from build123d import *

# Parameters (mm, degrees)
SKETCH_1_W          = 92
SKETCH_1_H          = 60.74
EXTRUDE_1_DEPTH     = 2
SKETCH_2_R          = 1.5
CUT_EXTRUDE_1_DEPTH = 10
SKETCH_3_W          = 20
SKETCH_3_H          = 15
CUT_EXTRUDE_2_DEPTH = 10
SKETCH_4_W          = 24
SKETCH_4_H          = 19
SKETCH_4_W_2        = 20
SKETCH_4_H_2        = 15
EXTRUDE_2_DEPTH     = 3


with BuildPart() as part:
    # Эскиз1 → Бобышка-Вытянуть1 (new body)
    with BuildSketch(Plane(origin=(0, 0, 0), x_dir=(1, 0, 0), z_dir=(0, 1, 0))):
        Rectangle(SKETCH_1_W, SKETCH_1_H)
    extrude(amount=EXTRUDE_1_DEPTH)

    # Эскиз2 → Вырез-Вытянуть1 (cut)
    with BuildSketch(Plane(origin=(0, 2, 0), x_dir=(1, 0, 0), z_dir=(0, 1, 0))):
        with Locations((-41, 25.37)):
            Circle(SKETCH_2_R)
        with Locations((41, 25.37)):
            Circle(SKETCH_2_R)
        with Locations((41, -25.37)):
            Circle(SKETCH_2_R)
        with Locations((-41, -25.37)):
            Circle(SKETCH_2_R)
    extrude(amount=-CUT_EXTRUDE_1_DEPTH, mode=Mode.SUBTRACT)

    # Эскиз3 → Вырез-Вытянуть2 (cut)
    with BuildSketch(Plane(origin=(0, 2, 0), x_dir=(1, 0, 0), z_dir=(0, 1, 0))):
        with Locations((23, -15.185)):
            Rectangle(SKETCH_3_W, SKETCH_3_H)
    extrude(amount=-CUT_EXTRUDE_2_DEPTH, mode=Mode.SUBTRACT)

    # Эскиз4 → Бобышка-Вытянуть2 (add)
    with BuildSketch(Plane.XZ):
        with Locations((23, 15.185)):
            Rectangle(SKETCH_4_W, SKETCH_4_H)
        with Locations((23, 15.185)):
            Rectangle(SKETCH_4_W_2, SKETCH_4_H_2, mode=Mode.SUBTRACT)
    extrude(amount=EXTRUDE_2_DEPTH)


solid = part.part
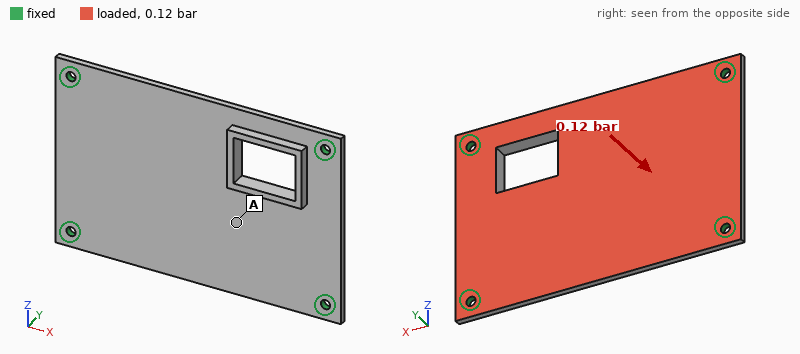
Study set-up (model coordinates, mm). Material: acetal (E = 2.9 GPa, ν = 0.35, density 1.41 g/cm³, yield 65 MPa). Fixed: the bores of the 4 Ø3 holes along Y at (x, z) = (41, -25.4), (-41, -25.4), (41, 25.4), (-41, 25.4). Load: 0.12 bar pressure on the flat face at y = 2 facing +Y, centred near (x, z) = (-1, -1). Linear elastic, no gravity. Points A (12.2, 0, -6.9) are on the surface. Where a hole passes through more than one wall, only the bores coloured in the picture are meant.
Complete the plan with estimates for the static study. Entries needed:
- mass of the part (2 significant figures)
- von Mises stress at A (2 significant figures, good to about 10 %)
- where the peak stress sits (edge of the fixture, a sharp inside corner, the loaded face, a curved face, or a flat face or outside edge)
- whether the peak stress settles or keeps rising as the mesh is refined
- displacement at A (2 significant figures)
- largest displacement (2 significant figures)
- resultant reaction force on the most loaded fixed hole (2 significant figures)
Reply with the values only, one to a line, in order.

15 g
3.8 MPa
edge of the fixture
keeps rising
0.85 mm
0.99 mm
17 N
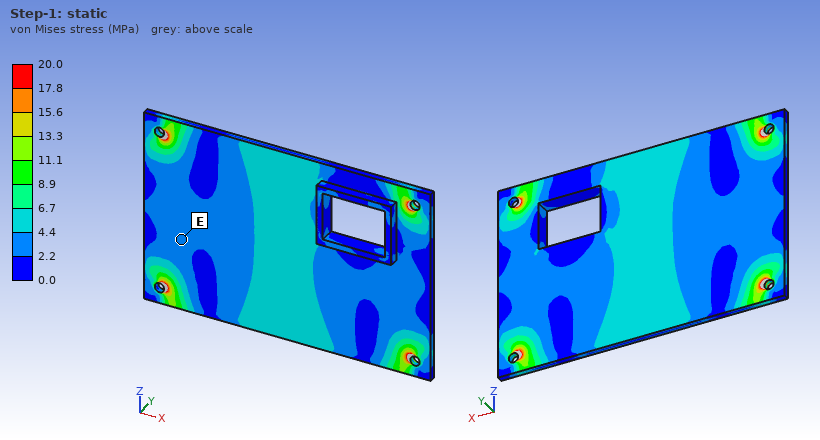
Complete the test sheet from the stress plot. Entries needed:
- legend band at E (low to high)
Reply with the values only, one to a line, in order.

2.2 to 4.4 MPa
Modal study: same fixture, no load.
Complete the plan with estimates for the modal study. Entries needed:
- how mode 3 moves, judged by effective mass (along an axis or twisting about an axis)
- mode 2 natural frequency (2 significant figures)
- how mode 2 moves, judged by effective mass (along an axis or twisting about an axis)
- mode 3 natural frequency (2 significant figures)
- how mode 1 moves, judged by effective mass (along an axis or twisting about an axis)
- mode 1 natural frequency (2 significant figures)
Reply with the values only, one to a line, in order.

twisting about Z
590 Hz
twisting about X
980 Hz
along Y
370 Hz
